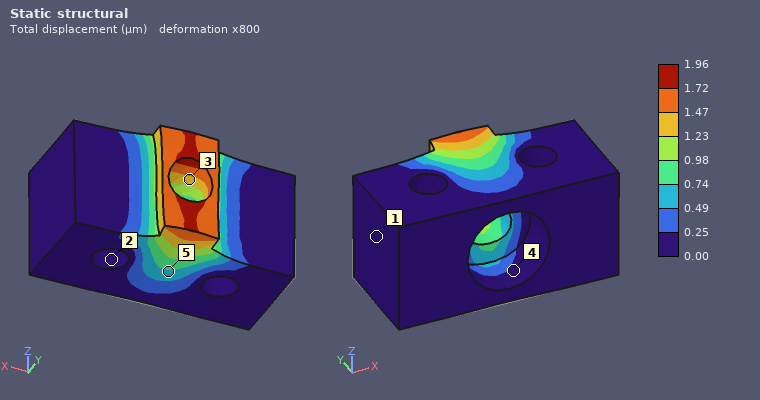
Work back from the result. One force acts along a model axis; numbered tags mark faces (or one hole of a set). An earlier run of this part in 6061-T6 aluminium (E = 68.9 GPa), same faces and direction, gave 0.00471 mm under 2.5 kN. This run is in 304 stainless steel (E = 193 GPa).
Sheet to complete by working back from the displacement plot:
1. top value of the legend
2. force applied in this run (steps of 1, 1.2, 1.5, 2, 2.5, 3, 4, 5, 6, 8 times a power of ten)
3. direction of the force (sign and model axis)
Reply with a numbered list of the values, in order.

1. 1.96 µm
2. 3 kN
3. +Z
